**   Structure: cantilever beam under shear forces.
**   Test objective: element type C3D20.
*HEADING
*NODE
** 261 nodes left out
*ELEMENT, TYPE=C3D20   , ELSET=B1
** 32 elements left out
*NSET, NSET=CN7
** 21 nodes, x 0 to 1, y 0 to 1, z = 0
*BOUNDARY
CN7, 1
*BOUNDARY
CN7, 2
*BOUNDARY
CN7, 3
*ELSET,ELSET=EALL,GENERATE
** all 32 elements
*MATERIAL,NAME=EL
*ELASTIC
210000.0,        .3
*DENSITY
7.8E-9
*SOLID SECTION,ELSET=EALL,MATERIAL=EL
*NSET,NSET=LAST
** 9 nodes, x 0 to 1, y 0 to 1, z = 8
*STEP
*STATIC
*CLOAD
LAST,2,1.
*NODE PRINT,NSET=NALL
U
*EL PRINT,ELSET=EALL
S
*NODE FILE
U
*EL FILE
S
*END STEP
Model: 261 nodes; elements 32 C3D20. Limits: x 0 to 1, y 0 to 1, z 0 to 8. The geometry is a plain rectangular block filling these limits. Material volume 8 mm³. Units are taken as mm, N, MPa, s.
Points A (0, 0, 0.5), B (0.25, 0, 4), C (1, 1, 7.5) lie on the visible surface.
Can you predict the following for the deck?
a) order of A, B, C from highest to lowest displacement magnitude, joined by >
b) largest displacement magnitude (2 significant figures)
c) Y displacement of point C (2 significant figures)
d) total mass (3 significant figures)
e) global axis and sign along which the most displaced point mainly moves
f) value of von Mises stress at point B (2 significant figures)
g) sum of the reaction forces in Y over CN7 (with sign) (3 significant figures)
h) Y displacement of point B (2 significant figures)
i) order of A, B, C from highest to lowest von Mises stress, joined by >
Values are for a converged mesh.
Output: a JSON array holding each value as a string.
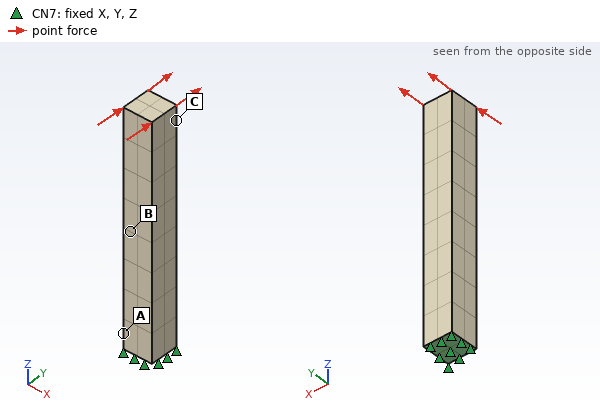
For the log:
["C > B > A", "0.089 mm", "0.080 mm", "6.24e-05 kg", "+Y", "220 MPa", "-9.00 N", "0.028 mm", "A > B > C"]
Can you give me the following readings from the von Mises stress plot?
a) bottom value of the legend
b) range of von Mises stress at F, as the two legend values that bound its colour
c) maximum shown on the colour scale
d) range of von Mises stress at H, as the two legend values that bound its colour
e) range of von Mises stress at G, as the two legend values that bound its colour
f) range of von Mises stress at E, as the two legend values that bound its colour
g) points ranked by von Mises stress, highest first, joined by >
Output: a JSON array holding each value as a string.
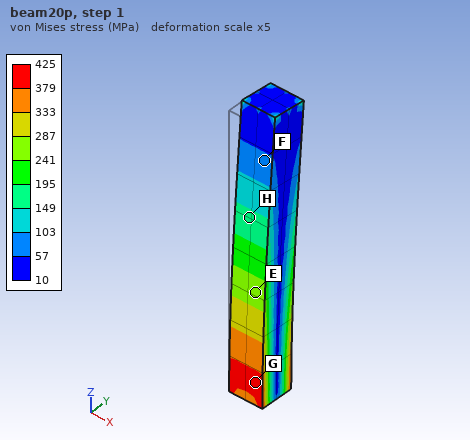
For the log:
["10 MPa", "57 to 103 MPa", "425 MPa", "149 to 195 MPa", "379 to 425 MPa", "241 to 287 MPa", "G > E > H > F"]
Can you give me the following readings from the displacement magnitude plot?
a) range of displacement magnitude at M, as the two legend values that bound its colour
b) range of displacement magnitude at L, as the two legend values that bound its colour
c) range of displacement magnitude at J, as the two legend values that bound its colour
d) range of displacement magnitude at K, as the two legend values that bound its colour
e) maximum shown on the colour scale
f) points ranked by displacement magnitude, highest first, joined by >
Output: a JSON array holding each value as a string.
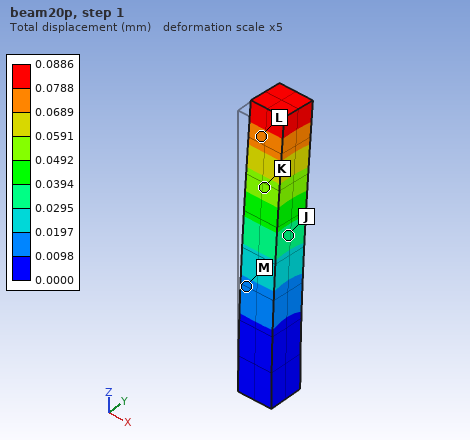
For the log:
["0.0098 to 0.0197 mm", "0.0689 to 0.0788 mm", "0.0295 to 0.0394 mm", "0.0492 to 0.0591 mm", "0.0886 mm", "L > K > J > M"]
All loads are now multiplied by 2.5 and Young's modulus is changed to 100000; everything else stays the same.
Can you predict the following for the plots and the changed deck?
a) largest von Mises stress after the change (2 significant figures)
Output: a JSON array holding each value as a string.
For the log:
["1100 MPa"]
